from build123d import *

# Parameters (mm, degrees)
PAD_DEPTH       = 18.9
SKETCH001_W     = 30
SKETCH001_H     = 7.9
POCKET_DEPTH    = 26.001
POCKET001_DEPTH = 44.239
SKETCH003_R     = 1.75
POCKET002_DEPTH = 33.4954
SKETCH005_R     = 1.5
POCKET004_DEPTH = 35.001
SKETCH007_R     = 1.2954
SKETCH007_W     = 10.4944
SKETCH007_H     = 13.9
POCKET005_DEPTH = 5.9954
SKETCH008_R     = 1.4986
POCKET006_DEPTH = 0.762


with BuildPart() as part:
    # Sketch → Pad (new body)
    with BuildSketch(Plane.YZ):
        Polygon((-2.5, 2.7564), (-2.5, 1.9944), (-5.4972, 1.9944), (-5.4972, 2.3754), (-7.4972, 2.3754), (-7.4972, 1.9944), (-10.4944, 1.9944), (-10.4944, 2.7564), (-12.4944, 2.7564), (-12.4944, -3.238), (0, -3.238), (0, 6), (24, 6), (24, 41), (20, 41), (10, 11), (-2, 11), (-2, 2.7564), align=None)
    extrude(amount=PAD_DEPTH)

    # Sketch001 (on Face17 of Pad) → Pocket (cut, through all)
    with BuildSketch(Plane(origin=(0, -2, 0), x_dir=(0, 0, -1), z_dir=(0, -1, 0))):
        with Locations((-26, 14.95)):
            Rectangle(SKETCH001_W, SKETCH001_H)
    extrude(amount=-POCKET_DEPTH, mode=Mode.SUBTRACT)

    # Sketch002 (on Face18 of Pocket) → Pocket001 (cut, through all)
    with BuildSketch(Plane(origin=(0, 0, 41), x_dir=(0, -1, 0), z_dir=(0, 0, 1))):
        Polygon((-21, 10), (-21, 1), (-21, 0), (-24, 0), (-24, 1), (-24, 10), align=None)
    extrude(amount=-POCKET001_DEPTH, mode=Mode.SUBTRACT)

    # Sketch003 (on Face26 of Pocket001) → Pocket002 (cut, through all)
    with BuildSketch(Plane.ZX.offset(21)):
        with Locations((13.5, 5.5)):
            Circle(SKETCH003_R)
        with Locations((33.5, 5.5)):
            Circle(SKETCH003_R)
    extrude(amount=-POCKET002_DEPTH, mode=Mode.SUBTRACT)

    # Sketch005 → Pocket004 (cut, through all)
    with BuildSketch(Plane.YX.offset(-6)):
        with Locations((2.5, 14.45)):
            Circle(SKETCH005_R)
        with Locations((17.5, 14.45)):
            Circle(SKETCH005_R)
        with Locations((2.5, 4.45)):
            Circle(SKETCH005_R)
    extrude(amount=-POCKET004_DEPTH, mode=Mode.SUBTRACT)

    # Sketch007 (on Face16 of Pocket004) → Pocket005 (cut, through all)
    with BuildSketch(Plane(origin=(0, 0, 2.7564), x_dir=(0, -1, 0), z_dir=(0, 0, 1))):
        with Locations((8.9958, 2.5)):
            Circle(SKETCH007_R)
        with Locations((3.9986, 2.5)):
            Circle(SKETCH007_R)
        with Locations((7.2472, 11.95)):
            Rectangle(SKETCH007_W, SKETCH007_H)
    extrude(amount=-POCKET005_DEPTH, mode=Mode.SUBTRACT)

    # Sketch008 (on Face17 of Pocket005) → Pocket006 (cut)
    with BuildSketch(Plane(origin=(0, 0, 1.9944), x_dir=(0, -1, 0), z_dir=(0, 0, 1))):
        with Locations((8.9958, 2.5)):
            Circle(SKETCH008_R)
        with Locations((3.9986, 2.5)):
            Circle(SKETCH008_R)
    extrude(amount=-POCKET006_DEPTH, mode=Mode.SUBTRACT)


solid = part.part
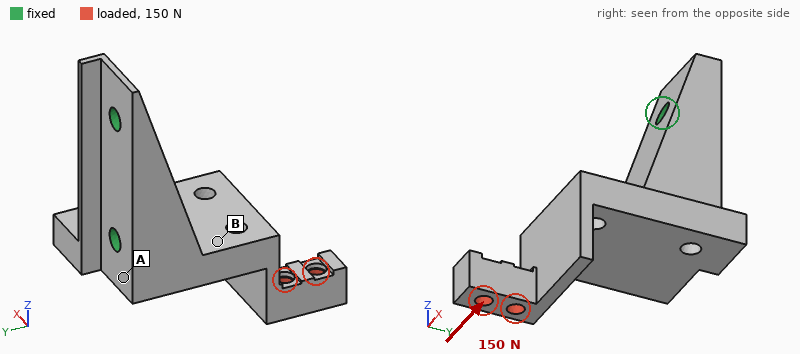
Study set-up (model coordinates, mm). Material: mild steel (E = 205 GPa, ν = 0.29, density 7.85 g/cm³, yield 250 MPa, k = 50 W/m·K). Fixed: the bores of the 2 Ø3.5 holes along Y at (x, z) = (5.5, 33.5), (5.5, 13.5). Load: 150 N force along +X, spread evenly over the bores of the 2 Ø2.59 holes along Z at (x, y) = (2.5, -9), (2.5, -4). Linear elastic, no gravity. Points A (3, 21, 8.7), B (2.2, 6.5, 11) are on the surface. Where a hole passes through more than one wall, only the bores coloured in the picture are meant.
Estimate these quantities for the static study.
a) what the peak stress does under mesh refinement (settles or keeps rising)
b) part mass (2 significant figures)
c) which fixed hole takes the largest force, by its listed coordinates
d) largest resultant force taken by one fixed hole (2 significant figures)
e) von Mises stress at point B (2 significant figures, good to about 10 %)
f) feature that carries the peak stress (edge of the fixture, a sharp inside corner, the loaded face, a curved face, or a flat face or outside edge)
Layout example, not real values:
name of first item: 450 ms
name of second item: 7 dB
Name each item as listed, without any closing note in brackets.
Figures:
what the peak stress does under mesh refinement: keeps rising
part mass: 37 g
which fixed hole takes the largest force, by its listed coordinates: (5.5, 13.5)
largest resultant force taken by one fixed hole: 190 N
von Mises stress at point B: 15 MPa
feature that carries the peak stress: a sharp inside corner
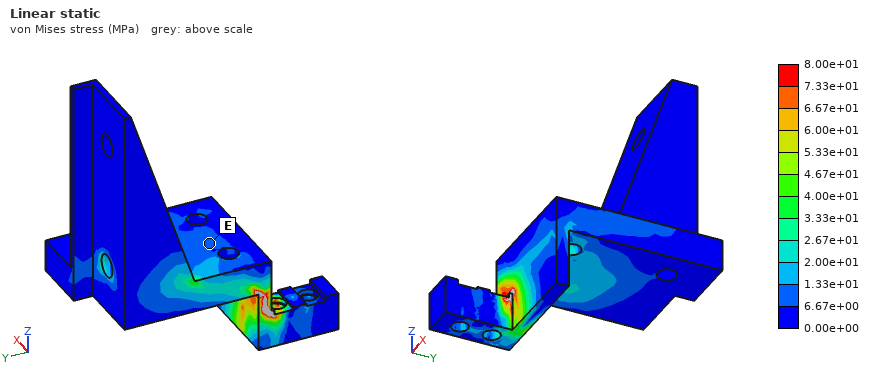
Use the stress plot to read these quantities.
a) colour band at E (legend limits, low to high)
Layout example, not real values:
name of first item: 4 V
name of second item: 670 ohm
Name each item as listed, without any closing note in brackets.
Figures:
colour band at E: 6.67e+00 to 1.33e+01 MPa
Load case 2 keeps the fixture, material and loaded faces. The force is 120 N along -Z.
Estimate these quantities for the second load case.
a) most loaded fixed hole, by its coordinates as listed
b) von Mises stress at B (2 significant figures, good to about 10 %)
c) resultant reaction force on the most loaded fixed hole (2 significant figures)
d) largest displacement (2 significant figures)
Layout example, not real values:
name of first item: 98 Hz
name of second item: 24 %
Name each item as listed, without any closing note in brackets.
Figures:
most loaded fixed hole, by its coordinates as listed: (5.5, 13.5)
von Mises stress at B: 29 MPa
resultant reaction force on the most loaded fixed hole: 130 N
largest displacement: 51 µm
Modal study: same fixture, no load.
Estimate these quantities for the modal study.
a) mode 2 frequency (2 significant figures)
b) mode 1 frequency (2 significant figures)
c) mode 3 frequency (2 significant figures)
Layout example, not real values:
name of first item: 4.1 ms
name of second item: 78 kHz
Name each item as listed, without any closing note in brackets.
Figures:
mode 2 frequency: 8300 Hz
mode 1 frequency: 5200 Hz
mode 3 frequency: 11 kHz
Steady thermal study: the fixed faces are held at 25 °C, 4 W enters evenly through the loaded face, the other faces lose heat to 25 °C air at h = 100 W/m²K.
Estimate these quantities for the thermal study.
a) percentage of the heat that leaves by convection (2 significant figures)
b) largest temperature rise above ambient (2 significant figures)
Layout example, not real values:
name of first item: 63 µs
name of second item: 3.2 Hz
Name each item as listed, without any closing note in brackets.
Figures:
percentage of the heat that leaves by convection: 52 %
largest temperature rise above ambient: 43 K
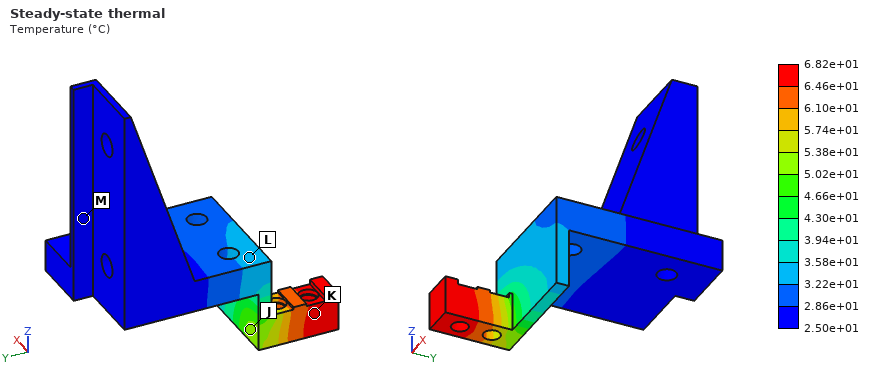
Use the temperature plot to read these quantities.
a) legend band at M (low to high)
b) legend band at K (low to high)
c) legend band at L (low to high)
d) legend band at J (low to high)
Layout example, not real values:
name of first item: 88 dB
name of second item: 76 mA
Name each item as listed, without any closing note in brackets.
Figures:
legend band at M: 2.50e+01 to 2.86e+01 °C
legend band at K: 6.46e+01 to 6.82e+01 °C
legend band at L: 3.22e+01 to 3.58e+01 °C
legend band at J: 5.02e+01 to 5.38e+01 °C
